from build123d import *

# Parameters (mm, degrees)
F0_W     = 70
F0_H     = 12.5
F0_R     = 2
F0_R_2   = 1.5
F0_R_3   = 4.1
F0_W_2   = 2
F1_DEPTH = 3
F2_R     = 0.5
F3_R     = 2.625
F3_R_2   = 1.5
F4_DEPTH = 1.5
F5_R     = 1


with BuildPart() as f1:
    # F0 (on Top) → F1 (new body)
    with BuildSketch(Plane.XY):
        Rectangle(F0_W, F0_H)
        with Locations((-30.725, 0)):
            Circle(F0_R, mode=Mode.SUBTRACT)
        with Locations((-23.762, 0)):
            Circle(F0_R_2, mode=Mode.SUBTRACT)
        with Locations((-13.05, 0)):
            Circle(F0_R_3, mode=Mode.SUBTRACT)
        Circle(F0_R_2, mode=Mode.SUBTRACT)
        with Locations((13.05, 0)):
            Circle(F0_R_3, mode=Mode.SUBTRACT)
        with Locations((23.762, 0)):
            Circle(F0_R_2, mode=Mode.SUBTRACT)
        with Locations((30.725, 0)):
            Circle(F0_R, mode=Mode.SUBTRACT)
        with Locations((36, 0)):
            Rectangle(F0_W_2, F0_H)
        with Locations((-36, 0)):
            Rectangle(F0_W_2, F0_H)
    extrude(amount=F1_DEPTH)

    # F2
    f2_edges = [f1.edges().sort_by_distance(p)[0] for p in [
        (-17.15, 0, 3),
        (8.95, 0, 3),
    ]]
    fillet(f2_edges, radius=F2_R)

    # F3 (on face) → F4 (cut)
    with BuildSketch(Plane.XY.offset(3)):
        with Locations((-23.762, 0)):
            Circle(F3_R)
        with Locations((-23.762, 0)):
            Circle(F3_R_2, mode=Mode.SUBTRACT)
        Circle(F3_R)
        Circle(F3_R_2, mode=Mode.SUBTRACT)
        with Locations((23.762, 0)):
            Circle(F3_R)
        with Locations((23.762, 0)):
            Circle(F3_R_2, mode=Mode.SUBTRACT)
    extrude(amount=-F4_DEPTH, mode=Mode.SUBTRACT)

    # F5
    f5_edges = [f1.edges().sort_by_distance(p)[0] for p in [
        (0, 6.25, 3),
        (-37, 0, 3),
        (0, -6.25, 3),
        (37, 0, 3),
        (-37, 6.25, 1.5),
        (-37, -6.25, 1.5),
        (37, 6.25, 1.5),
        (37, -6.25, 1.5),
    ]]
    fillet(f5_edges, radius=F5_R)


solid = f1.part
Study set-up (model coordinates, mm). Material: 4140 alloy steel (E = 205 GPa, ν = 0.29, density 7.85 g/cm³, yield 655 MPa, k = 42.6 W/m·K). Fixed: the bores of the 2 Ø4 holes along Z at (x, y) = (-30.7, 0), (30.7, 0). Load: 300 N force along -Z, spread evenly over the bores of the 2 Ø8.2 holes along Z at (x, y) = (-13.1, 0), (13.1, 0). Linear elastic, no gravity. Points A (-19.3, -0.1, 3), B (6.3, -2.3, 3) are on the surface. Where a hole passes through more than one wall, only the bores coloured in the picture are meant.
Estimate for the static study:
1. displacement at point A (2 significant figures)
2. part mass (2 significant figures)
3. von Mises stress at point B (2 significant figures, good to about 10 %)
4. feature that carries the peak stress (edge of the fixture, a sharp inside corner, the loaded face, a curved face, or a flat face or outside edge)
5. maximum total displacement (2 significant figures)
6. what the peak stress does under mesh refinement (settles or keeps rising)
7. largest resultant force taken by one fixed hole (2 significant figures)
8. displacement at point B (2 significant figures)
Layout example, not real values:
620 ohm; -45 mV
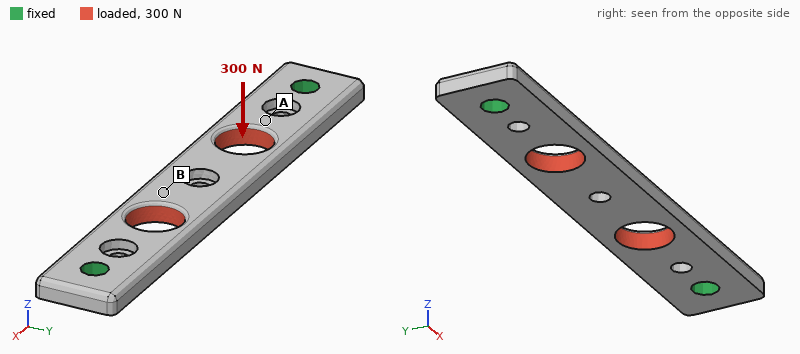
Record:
18 µm; 17 g; 30 MPa; edge of the fixture; 47 µm; keeps rising; 150 N; 44 µm
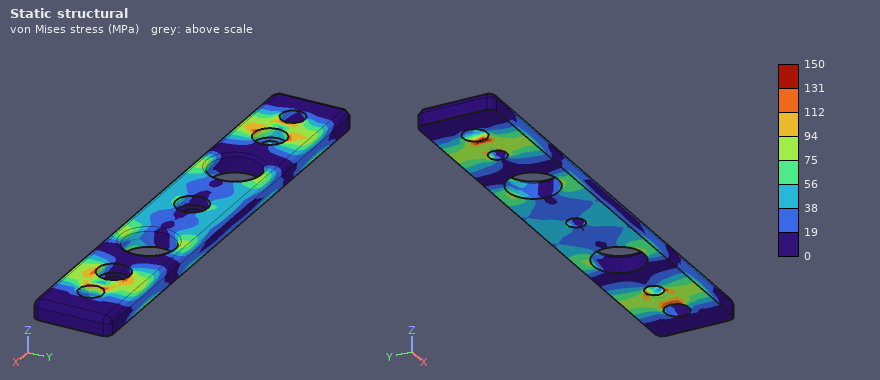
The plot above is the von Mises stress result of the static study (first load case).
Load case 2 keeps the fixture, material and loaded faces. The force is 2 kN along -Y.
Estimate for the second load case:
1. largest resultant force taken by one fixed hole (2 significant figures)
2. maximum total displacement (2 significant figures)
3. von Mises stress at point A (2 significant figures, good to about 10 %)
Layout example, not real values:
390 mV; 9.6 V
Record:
1.0 kN; 51 µm; 140 MPa
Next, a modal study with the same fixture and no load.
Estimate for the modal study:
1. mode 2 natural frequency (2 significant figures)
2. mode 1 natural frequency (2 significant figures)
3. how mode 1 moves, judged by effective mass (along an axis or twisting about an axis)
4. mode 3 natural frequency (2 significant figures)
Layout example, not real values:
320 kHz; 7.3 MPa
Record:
9900 Hz; 4200 Hz; along Z; 10 kHz
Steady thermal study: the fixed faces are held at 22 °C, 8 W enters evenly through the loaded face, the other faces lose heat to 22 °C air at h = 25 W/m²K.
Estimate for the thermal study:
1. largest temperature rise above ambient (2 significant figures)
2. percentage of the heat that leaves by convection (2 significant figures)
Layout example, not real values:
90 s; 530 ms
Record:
56 K; 18 %
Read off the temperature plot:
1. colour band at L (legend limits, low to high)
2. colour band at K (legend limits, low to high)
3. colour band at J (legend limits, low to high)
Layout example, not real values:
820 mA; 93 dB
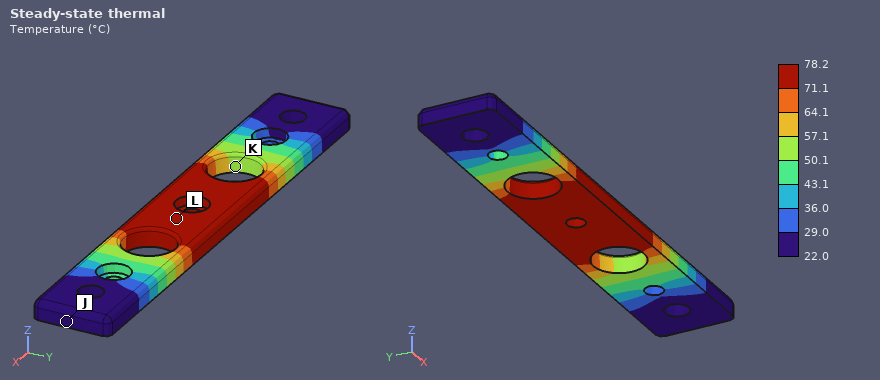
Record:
71.1 to 78.2 °C; 50.1 to 57.1 °C; 22.0 to 29.0 °C
